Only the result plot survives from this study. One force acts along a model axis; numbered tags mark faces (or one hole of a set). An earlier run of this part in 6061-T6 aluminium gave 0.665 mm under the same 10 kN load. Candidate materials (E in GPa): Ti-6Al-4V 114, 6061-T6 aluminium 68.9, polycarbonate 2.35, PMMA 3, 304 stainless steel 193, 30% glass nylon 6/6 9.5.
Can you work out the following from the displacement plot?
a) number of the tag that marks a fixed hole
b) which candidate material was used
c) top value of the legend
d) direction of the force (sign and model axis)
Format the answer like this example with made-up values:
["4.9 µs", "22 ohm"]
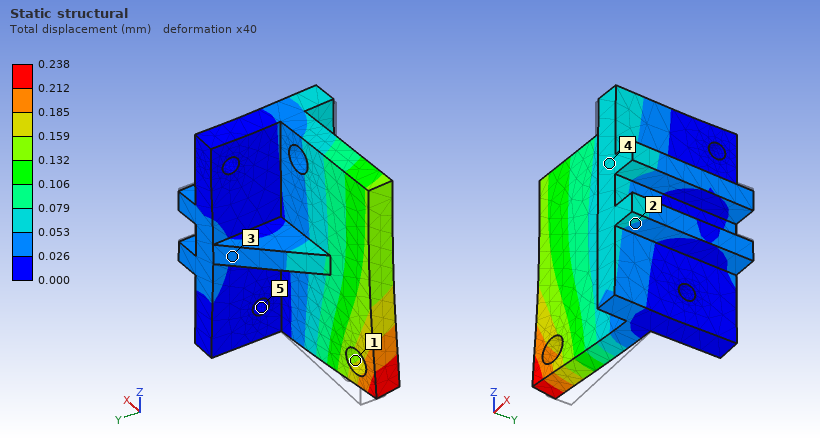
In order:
["5", "304 stainless steel", "0.238 mm", "-Y"]
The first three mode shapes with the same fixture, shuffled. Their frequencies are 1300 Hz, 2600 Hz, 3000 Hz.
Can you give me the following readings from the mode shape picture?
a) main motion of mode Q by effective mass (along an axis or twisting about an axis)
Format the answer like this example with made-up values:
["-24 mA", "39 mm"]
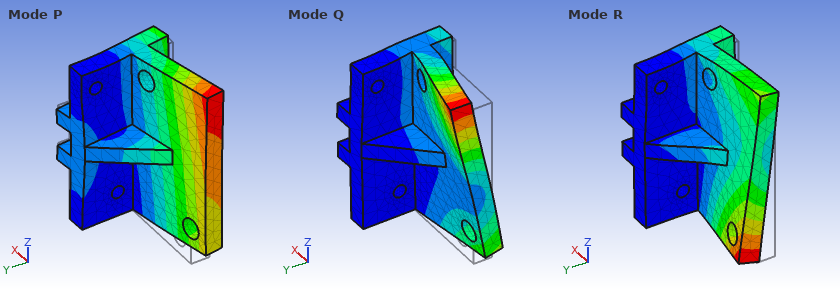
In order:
["along X"]
